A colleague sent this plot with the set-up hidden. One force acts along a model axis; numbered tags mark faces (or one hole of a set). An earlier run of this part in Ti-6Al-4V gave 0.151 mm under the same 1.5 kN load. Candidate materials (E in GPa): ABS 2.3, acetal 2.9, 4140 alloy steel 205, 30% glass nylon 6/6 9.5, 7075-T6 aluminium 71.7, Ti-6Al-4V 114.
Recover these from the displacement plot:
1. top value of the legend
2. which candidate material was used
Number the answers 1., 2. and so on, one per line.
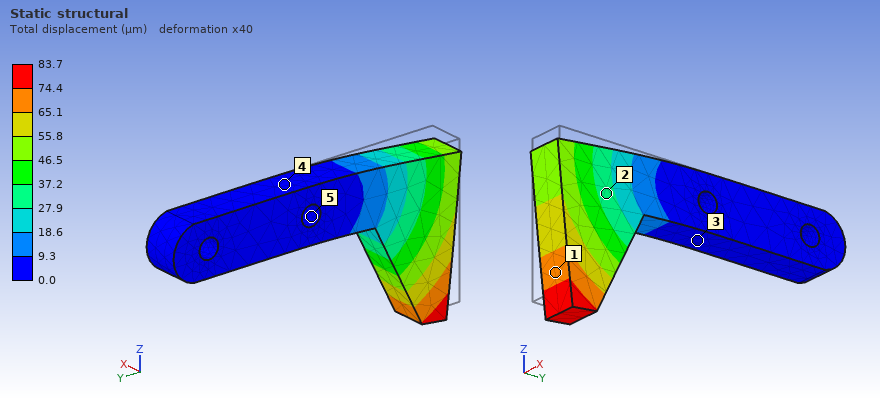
1. 83.7 µm
2. 4140 alloy steel
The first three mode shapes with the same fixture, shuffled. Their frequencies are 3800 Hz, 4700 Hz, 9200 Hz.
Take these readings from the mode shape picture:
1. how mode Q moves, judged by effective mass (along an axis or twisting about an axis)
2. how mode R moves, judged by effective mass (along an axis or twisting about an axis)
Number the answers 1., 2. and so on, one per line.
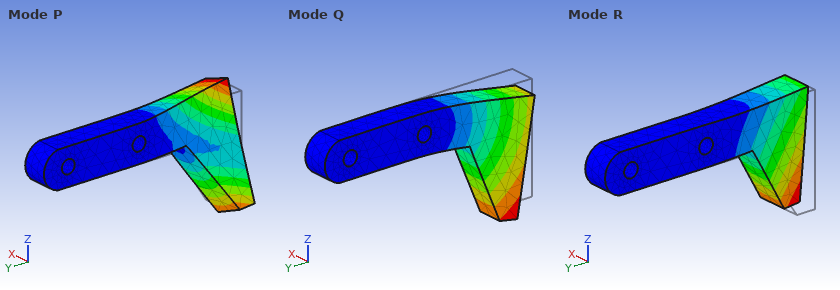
1. along Z
2. along X
